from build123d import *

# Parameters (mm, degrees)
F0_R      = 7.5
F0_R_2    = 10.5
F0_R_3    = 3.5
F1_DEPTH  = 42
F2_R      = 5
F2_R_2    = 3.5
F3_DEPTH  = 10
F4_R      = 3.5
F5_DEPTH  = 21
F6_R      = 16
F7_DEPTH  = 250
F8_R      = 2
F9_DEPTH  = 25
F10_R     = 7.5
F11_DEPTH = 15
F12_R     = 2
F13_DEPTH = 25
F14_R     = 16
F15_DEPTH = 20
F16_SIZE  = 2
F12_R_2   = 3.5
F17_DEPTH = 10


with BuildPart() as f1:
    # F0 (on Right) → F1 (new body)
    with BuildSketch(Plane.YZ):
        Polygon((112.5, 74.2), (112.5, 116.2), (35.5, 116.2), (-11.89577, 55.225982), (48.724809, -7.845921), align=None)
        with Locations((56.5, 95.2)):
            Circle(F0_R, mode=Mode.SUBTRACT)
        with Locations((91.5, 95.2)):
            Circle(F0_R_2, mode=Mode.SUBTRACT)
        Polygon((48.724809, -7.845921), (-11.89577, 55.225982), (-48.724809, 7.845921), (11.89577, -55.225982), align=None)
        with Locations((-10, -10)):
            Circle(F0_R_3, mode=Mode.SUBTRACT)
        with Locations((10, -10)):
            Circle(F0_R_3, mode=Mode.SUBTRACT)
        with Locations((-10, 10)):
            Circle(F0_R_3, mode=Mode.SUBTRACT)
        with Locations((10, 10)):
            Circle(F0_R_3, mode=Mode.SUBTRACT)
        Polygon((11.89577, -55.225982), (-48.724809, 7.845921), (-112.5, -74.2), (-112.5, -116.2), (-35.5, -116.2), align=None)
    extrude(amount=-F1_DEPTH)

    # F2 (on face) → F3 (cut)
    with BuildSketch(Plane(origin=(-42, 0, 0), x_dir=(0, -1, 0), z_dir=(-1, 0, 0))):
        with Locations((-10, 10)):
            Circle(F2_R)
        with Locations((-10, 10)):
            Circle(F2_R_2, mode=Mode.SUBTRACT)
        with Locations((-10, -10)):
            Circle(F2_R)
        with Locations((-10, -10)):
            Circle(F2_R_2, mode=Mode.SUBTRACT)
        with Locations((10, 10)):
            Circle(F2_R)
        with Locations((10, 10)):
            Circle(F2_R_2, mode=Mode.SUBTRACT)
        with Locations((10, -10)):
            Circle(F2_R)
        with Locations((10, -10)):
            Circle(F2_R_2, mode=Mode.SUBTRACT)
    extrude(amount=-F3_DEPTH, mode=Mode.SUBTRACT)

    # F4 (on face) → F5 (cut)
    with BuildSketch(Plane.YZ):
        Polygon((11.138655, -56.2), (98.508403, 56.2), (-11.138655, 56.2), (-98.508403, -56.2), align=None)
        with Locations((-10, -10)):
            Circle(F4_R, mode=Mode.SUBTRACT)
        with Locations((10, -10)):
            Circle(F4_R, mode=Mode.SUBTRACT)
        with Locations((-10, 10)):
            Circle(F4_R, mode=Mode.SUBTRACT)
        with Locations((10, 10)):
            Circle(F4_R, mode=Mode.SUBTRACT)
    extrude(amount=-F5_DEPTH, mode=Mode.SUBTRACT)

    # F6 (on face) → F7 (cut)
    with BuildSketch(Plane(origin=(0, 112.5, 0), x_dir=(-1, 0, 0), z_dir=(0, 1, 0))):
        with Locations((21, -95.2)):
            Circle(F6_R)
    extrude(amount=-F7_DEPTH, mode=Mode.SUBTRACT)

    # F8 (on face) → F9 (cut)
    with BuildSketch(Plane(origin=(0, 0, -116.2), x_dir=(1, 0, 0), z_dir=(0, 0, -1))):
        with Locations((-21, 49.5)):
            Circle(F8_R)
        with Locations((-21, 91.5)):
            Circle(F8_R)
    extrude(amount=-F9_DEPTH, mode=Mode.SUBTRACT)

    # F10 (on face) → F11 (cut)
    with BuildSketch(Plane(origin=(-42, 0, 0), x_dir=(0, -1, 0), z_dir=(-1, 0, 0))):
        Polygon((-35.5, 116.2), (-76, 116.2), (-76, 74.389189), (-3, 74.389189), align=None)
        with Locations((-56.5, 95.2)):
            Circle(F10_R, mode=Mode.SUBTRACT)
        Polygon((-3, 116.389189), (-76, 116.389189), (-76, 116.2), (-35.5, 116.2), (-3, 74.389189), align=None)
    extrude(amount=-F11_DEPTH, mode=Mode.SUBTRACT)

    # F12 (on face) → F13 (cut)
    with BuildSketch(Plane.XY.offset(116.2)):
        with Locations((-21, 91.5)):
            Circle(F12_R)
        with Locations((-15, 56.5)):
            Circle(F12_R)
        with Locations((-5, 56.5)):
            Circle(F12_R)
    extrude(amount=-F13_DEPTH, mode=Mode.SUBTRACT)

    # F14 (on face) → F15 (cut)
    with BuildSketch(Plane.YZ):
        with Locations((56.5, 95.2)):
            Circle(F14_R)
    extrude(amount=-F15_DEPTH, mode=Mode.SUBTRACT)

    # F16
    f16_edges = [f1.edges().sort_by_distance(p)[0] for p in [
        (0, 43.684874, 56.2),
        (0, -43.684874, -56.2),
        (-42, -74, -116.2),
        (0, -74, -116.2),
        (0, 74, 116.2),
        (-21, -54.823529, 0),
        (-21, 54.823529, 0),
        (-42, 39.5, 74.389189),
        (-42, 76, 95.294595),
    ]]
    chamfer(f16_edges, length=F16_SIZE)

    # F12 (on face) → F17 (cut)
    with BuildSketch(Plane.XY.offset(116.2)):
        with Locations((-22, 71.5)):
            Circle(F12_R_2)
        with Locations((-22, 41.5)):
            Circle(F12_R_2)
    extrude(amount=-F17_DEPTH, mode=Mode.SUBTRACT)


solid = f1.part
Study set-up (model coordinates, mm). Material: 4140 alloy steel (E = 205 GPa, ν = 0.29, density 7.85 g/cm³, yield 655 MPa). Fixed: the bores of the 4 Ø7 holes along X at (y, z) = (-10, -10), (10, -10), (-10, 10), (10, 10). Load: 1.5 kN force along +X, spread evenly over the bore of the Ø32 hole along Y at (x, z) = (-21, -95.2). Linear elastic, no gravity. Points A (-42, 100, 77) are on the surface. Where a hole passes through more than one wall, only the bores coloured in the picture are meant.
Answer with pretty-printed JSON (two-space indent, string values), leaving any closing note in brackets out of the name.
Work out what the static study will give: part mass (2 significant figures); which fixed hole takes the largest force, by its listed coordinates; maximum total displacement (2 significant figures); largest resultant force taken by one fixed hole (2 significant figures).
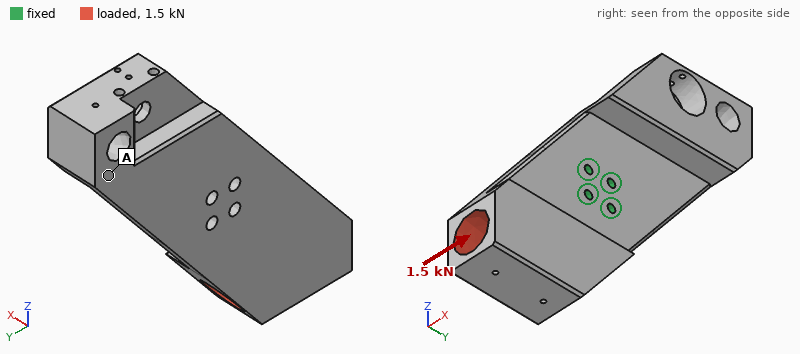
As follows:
{
  "part mass": "4.7 kg",
  "which fixed hole takes the largest force, by its listed coordinates": "(-10, -10)",
  "maximum total displacement": "87 µm",
  "largest resultant force taken by one fixed hole": "5.3 kN"
}
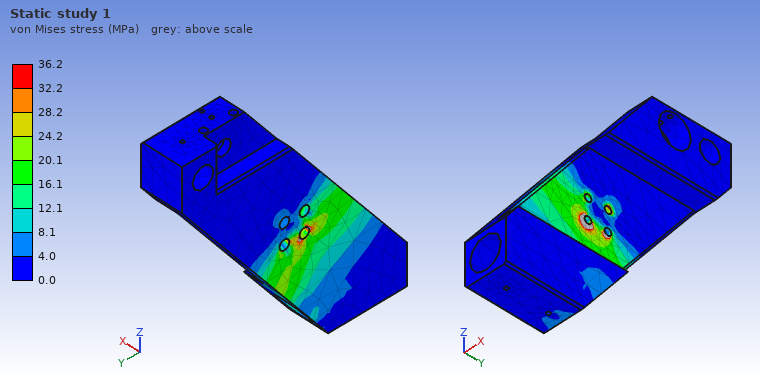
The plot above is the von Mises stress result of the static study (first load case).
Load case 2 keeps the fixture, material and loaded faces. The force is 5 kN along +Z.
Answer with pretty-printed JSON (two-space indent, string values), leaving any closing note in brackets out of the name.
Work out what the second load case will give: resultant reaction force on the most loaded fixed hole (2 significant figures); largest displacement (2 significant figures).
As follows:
{
  "resultant reaction force on the most loaded fixed hole": "6.6 kN",
  "largest displacement": "39 µm"
}
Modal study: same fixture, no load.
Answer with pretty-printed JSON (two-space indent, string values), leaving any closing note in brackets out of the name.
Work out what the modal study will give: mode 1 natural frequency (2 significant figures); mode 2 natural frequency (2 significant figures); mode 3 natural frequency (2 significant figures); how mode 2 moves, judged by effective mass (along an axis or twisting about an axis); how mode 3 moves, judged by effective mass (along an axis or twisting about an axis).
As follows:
{
  "mode 1 natural frequency": "700 Hz",
  "mode 2 natural frequency": "810 Hz",
  "mode 3 natural frequency": "1500 Hz",
  "how mode 2 moves, judged by effective mass": "along X",
  "how mode 3 moves, judged by effective mass": "twisting about X"
}
